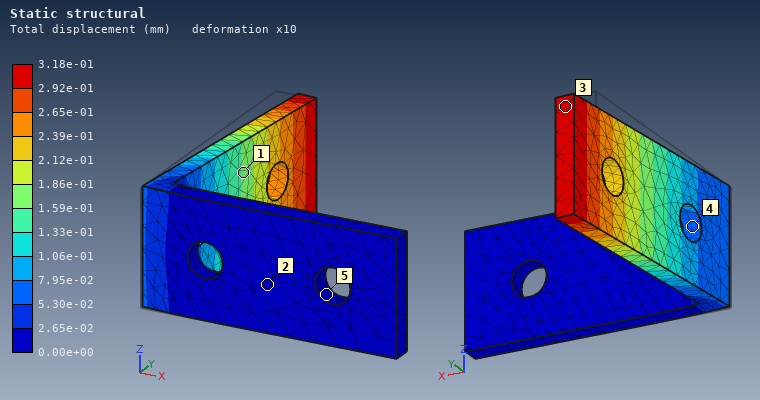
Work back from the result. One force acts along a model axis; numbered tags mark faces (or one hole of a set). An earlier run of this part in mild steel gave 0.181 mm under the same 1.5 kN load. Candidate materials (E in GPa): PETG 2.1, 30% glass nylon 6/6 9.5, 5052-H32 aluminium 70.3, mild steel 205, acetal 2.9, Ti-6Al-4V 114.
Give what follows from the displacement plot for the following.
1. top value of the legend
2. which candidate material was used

3.18e-01 mm
Ti-6Al-4V
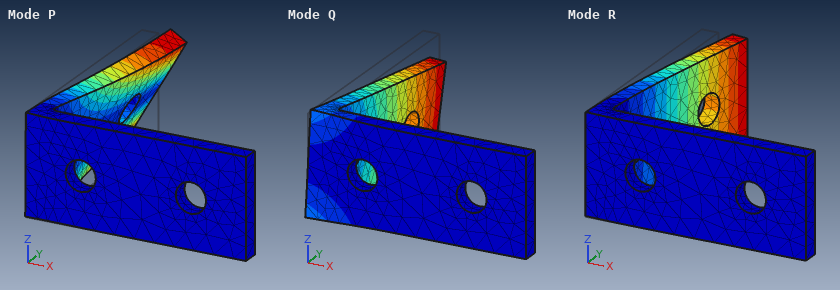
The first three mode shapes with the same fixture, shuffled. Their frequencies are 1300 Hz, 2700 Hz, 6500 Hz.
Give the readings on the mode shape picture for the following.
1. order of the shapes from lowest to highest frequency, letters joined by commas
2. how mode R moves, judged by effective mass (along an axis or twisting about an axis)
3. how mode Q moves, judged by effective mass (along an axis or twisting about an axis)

R, Q, P
along X
along Z
